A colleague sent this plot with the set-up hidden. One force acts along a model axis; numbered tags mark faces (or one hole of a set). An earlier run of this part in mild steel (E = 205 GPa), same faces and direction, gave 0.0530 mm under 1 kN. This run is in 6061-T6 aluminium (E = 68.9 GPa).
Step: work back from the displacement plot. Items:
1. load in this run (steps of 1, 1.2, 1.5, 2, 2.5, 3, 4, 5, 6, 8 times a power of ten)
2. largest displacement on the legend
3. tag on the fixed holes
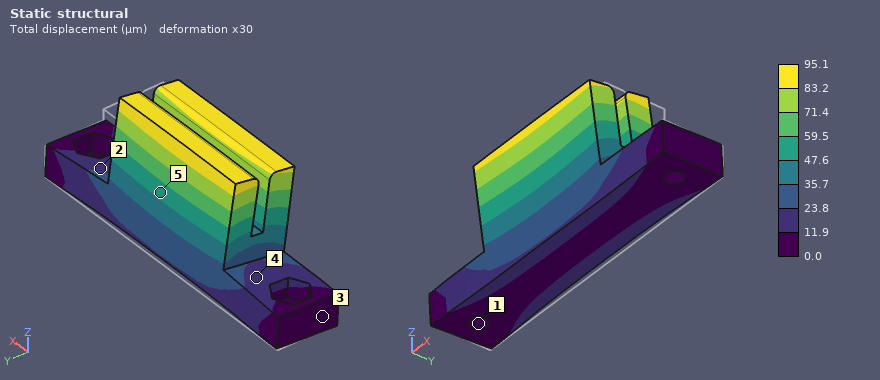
600 N
95.1 µm
1
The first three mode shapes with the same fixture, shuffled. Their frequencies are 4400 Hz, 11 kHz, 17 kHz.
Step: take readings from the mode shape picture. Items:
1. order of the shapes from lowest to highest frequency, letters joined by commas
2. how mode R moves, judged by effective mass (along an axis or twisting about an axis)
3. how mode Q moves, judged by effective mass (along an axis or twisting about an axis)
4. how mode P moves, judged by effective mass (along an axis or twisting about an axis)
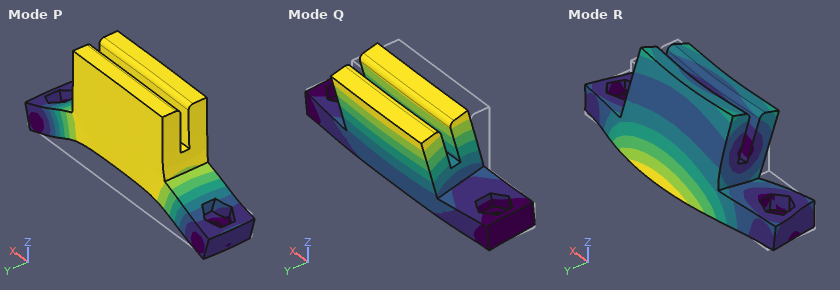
Q, P, R
along Y
along Y
along Z
